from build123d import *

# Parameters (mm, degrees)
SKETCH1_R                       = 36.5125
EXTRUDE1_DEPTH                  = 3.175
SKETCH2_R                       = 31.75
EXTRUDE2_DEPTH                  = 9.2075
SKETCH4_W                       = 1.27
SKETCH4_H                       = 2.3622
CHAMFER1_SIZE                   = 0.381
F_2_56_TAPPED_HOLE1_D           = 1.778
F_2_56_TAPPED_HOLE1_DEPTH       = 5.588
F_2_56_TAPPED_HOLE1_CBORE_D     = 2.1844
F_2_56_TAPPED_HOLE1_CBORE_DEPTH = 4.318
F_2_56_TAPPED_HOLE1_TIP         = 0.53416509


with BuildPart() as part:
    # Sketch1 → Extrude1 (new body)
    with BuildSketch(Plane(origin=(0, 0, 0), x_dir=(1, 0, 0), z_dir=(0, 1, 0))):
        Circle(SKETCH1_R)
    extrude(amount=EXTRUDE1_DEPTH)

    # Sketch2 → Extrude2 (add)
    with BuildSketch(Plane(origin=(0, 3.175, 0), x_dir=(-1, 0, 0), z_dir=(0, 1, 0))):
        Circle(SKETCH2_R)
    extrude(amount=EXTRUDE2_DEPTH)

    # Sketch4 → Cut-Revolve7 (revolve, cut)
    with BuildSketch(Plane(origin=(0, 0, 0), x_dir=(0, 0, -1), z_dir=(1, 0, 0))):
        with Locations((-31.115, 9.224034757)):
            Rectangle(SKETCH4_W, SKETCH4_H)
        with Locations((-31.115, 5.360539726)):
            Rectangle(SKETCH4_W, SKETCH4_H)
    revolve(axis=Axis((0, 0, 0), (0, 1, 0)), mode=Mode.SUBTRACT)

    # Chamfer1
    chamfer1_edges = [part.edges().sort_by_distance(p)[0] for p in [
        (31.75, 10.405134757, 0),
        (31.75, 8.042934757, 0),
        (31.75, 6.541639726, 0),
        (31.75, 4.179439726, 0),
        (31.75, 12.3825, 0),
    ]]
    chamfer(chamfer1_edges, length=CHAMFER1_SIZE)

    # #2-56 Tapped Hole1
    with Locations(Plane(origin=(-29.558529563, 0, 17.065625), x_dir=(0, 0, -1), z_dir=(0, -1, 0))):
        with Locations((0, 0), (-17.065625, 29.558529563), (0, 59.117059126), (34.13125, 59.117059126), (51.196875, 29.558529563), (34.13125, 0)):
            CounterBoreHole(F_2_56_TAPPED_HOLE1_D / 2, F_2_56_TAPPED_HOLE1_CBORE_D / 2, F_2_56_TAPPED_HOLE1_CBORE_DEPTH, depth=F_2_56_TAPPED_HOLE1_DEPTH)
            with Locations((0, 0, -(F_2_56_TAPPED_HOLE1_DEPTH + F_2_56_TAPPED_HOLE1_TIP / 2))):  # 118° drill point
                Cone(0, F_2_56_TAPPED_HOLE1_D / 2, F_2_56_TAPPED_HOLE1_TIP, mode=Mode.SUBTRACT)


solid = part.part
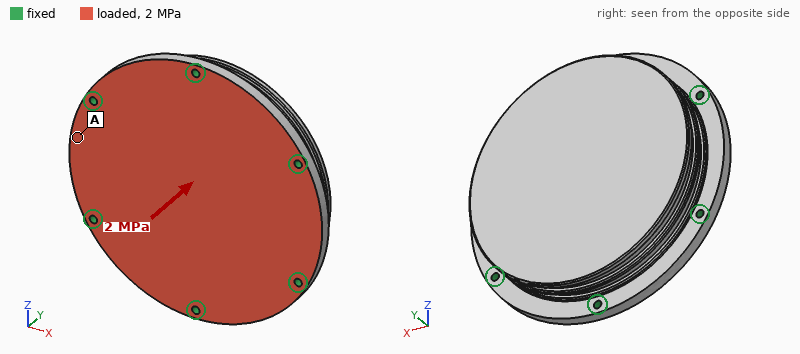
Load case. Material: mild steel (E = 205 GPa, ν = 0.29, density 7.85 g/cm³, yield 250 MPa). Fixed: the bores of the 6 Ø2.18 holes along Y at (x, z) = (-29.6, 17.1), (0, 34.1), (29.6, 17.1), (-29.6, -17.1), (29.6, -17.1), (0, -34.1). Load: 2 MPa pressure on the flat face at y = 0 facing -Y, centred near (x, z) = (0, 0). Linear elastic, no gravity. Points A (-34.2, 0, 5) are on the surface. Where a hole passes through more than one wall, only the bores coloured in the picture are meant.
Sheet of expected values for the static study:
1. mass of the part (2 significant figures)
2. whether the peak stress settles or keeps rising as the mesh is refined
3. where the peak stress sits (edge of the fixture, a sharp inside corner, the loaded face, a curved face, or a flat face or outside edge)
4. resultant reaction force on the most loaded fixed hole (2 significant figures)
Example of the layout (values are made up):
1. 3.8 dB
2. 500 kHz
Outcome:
1. 320 g
2. keeps rising
3. edge of the fixture
4. 1.6 kN
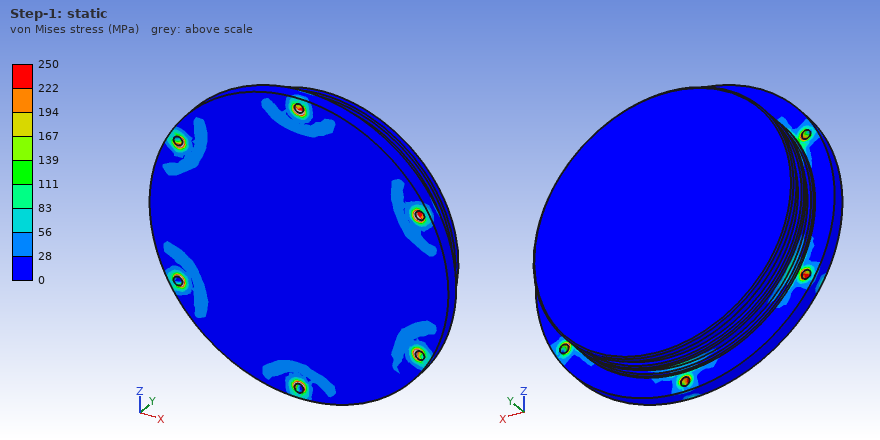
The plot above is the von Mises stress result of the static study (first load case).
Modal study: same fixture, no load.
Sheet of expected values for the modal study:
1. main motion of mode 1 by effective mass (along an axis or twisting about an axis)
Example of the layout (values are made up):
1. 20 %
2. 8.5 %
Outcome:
1. along Y
